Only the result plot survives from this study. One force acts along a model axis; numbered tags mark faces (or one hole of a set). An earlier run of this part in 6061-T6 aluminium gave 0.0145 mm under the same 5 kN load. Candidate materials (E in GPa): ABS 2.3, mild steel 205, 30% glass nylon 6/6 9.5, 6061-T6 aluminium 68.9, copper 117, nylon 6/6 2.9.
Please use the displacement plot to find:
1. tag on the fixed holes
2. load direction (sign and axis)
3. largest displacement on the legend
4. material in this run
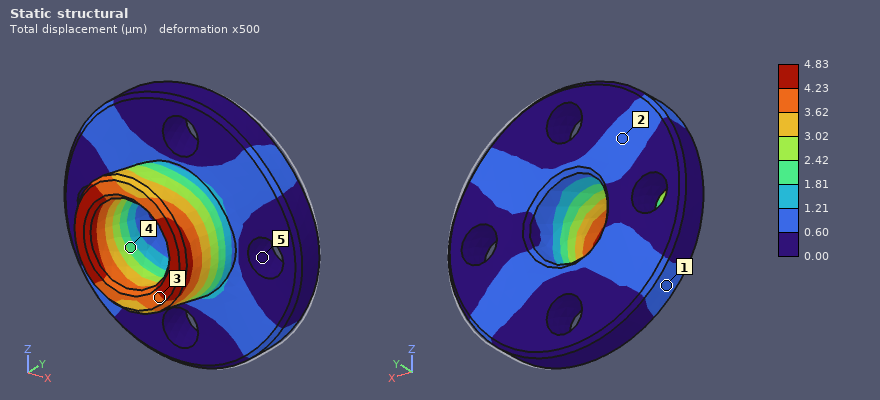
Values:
5
-X
4.83 µm
mild steel
